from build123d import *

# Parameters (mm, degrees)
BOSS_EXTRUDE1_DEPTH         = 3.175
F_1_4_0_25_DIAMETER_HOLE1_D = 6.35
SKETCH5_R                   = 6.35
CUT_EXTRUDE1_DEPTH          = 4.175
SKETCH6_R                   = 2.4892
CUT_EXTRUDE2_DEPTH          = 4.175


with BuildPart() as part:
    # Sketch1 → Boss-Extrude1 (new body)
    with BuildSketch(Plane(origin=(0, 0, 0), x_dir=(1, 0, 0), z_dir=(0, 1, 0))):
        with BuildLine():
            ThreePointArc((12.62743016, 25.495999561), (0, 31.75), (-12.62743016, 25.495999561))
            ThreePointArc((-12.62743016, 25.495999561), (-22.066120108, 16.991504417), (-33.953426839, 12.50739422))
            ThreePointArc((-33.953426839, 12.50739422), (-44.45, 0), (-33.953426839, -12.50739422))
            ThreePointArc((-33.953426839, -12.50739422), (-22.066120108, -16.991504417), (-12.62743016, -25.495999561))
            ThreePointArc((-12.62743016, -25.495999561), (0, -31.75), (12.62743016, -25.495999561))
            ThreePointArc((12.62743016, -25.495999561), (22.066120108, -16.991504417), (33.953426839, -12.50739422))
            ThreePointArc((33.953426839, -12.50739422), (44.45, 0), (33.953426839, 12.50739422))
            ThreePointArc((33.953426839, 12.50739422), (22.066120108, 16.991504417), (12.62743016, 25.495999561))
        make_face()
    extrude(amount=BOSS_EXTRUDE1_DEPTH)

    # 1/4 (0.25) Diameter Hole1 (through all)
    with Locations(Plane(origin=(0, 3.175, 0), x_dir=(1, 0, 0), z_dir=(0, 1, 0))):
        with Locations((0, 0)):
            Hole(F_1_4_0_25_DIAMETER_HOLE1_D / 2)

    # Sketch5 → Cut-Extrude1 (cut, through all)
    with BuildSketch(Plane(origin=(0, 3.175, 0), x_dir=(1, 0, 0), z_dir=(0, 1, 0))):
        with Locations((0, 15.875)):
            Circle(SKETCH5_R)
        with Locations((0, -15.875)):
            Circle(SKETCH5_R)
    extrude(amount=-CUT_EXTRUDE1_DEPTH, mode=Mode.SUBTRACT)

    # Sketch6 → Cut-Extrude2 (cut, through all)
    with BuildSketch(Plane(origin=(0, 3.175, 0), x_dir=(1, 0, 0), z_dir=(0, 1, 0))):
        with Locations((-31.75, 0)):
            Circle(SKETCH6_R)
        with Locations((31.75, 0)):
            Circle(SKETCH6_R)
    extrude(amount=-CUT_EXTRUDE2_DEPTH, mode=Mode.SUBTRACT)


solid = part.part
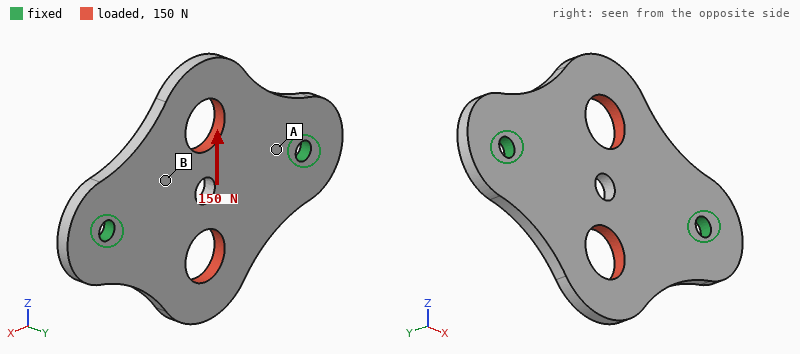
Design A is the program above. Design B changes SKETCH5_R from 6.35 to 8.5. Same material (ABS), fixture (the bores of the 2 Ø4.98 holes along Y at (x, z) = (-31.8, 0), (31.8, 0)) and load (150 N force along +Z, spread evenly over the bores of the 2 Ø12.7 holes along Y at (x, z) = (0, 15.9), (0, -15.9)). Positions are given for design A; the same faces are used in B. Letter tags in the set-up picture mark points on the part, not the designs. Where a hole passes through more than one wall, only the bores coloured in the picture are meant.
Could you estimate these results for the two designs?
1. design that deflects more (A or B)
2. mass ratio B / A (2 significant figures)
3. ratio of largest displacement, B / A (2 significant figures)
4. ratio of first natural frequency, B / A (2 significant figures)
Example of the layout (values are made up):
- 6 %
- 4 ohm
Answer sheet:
- B
- 0.93
- 1.3
- 1.0
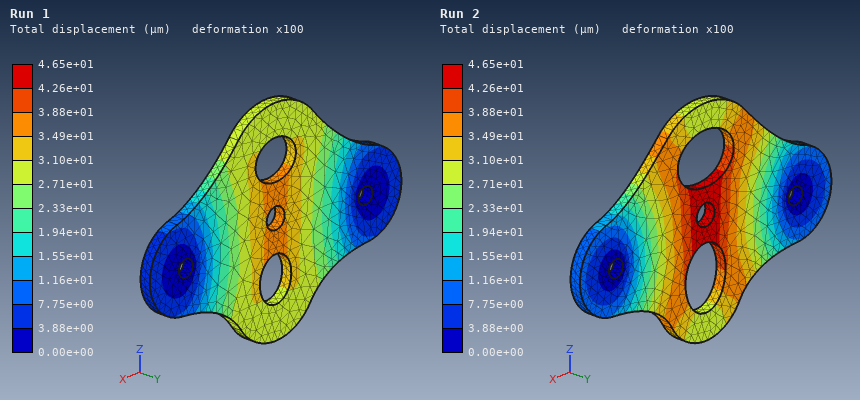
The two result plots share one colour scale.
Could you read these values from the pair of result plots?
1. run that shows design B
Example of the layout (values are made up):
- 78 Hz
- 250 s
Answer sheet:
- Run 2
